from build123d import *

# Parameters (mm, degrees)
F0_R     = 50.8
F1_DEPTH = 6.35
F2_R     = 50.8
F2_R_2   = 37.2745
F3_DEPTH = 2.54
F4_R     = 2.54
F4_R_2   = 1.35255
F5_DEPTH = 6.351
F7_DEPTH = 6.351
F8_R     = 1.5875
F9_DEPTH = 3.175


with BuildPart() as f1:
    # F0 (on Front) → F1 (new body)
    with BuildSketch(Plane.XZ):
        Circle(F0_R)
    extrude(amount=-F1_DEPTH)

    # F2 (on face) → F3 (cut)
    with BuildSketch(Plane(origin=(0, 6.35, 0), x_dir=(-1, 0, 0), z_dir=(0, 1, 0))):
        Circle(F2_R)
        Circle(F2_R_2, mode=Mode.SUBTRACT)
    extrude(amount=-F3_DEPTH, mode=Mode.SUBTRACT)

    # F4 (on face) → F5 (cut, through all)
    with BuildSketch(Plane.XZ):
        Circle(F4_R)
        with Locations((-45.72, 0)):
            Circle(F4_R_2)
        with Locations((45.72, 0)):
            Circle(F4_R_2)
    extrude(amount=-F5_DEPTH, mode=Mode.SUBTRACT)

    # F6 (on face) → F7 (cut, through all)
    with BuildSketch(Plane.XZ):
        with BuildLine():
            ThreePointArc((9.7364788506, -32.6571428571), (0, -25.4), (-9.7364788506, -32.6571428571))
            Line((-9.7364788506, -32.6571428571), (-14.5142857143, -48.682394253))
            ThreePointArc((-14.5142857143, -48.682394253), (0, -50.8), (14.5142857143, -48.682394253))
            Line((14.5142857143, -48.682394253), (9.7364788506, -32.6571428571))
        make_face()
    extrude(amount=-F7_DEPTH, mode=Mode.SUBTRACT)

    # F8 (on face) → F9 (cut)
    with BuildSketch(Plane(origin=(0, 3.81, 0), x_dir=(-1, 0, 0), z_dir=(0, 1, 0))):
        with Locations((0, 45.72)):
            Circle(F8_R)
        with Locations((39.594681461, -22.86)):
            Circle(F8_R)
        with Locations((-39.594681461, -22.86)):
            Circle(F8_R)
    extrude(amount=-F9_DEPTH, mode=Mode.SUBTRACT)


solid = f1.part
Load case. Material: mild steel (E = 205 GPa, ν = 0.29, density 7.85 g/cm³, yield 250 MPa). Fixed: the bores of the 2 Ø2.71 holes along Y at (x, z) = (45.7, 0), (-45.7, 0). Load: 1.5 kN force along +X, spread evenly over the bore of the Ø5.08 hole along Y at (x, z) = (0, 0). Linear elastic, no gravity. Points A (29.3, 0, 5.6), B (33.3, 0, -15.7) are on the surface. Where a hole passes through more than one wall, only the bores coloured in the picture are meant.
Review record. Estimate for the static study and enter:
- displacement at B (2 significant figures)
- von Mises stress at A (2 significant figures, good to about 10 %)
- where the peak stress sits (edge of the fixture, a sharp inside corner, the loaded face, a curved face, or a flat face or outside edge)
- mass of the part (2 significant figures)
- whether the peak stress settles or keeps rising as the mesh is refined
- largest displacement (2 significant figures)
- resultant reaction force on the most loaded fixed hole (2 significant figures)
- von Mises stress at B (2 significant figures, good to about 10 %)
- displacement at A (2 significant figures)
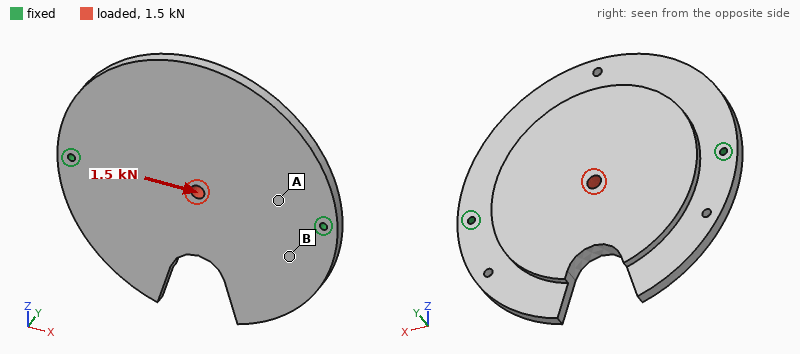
1.1 µm
6.9 MPa
edge of the fixture
310 g
keeps rising
2.0 µm
750 N
3.2 MPa
1.0 µm
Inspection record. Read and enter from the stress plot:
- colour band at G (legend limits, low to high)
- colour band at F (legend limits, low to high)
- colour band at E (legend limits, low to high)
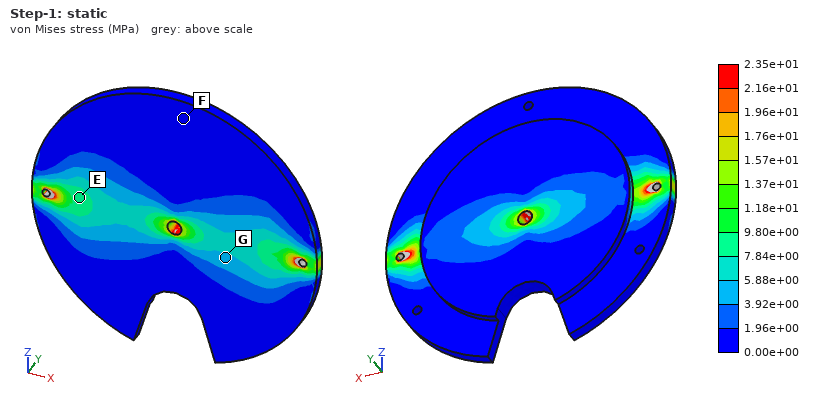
3.92e+00 to 5.88e+00 MPa
0.00e+00 to 1.96e+00 MPa
7.84e+00 to 9.80e+00 MPa
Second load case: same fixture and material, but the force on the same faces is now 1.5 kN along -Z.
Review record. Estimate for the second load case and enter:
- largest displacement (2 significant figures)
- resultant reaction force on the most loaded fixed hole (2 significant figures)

18 µm
750 N
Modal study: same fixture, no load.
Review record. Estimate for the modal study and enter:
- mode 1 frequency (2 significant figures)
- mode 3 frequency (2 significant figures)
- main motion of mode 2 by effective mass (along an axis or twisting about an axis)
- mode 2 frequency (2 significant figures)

930 Hz
3500 Hz
along Y
1700 Hz
